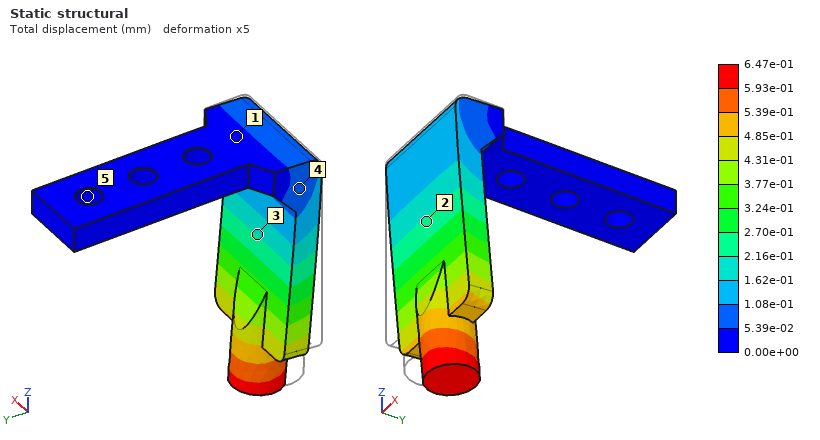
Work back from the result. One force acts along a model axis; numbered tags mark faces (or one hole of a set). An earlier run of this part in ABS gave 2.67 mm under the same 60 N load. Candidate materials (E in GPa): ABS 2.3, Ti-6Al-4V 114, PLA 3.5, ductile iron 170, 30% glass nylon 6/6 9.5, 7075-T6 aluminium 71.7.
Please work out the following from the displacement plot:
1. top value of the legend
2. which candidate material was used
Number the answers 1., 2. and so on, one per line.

1. 6.47e-01 mm
2. 30% glass nylon 6/6
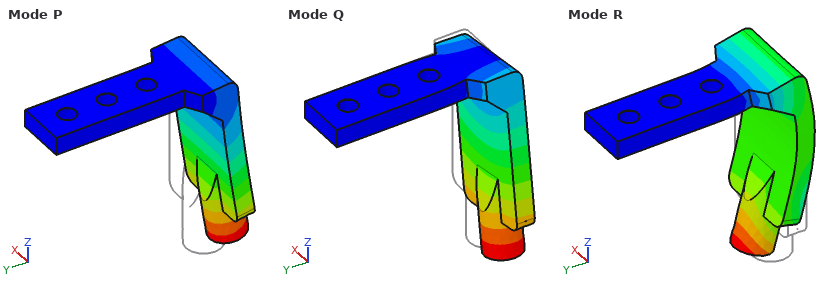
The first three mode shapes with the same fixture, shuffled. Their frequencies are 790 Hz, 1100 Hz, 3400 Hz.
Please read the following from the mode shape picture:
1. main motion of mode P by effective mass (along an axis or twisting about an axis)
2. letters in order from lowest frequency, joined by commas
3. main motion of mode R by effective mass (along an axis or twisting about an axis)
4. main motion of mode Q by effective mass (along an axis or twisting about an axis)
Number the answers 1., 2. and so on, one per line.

1. along Y
2. P, Q, R
3. along Z
4. along X
